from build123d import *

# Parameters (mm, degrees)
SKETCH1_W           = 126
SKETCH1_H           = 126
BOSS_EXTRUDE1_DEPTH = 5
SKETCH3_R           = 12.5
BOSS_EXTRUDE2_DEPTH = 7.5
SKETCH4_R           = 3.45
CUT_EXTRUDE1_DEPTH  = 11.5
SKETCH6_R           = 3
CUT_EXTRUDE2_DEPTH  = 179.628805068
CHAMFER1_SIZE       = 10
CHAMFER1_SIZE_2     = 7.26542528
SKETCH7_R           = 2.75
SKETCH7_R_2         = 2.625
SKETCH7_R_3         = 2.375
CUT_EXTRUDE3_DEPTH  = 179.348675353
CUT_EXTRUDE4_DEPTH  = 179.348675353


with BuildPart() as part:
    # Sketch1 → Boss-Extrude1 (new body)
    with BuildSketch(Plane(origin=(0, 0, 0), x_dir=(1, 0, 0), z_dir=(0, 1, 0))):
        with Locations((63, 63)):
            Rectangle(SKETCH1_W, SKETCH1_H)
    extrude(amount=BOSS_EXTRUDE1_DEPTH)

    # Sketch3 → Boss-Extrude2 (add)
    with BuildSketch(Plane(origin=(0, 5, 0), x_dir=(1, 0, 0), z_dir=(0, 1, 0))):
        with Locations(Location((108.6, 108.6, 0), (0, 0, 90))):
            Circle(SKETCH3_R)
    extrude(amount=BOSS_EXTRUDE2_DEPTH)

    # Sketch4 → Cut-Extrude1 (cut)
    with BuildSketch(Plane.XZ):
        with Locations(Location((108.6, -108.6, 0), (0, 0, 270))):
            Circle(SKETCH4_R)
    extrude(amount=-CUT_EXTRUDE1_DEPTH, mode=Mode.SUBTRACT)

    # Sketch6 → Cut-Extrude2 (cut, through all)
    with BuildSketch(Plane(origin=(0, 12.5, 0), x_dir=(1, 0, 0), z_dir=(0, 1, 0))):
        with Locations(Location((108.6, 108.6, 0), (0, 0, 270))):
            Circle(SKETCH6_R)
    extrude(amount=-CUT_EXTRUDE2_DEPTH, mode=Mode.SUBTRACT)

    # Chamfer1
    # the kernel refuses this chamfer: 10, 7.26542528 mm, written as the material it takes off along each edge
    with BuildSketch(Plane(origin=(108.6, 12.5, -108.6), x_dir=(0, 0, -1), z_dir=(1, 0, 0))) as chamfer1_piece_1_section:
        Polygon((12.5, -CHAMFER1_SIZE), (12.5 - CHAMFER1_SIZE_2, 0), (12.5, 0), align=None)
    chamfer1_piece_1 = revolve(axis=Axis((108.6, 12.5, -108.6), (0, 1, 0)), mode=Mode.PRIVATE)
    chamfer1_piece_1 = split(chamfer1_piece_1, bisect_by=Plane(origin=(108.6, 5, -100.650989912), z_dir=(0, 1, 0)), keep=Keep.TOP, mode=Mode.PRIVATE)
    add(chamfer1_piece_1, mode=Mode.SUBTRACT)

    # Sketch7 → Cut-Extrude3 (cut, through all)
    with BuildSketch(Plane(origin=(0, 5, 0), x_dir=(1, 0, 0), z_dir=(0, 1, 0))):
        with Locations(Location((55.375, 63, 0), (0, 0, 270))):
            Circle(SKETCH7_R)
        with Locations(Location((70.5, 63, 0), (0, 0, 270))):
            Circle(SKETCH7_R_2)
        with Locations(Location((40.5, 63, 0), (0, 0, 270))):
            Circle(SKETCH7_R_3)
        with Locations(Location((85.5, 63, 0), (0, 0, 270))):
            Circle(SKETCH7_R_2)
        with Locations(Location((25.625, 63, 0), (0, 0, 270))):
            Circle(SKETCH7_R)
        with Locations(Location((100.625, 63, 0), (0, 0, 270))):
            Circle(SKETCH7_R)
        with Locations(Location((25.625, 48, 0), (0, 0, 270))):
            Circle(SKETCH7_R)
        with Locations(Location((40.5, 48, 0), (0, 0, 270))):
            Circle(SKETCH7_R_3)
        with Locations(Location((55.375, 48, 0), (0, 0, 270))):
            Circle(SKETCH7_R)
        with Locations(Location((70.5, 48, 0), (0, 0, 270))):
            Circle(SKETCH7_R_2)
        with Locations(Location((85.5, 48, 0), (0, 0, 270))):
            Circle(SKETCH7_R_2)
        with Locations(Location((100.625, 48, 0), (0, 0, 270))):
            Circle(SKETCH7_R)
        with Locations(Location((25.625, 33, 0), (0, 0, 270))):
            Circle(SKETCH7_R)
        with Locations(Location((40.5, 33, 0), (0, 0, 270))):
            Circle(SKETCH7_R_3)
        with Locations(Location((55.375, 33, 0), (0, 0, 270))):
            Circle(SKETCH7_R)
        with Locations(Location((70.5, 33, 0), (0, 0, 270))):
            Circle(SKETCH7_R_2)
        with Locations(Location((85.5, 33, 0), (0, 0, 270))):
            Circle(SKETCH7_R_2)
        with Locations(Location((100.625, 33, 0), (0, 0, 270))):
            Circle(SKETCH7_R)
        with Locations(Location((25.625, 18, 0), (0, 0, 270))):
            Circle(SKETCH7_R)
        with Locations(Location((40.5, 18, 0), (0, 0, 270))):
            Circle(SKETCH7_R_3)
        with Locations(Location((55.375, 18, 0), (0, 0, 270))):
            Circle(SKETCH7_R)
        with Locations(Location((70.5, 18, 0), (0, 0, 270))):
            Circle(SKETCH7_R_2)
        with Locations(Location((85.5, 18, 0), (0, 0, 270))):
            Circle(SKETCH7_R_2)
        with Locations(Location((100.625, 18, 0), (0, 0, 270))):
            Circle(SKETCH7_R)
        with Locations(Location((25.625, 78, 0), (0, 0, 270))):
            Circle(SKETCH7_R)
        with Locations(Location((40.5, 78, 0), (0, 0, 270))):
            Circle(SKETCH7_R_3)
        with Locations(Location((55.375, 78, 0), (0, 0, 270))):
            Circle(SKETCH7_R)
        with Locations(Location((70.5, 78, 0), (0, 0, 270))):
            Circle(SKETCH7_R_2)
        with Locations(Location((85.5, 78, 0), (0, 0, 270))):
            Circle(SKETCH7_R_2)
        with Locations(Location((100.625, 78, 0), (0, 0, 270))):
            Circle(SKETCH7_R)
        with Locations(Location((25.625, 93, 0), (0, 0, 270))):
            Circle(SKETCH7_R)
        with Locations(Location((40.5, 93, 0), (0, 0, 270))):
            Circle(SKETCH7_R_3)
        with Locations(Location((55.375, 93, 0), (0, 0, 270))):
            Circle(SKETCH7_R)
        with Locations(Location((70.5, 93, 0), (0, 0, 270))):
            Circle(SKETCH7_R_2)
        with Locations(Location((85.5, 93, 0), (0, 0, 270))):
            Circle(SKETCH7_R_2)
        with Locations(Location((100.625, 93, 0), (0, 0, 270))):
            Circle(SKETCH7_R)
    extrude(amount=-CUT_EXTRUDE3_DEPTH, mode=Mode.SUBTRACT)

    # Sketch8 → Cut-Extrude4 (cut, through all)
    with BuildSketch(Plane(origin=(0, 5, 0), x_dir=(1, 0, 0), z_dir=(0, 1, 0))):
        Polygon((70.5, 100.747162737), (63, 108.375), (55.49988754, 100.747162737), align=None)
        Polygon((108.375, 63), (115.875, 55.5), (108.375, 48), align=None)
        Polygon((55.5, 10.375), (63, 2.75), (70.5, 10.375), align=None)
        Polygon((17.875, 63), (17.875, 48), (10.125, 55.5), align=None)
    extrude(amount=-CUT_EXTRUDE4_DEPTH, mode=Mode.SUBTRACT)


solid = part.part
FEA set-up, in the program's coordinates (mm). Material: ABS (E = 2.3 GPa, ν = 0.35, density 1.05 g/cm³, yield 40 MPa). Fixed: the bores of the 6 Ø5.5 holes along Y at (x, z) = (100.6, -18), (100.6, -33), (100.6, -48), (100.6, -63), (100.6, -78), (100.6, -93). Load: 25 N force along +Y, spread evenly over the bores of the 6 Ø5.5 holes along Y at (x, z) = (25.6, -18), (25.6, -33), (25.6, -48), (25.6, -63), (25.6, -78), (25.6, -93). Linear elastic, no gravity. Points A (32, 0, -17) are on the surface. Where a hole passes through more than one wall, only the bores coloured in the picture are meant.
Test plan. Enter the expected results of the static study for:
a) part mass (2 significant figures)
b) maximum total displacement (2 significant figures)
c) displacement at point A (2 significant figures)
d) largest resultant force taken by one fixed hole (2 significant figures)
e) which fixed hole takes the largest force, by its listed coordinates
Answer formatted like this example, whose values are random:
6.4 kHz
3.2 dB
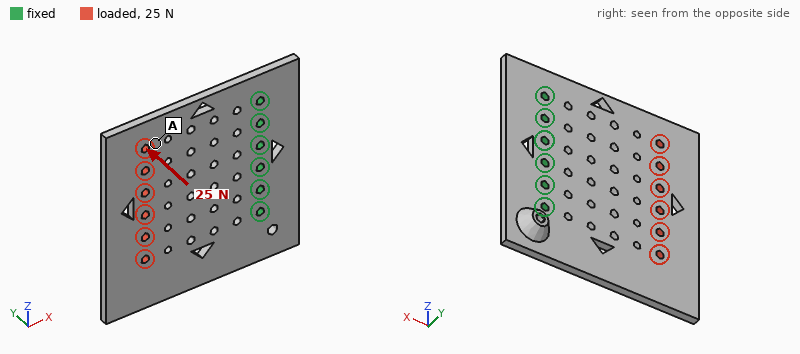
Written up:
79 g
2.0 mm
1.1 mm
6.6 N
(100.6, -33)
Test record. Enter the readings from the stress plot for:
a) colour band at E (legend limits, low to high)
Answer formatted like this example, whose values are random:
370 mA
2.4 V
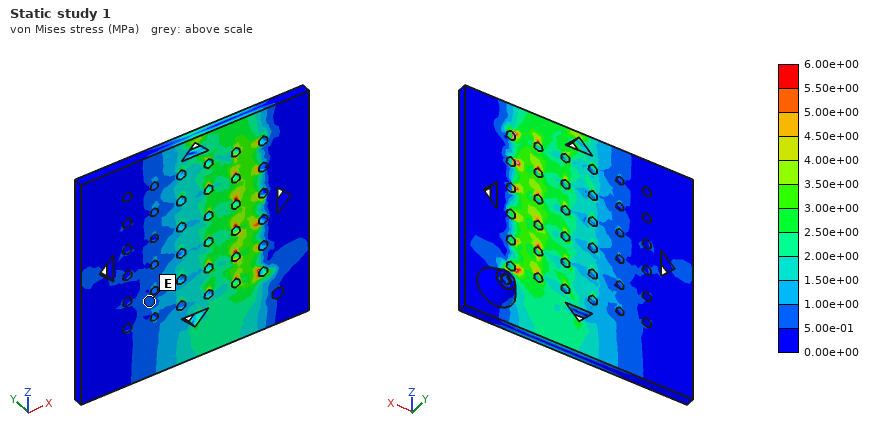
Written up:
5.00e-01 to 1.00e+00 MPa
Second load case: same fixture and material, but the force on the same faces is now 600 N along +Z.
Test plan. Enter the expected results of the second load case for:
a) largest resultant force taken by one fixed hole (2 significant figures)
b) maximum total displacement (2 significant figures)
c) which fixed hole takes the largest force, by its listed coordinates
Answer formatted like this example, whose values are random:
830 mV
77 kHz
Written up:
550 N
0.32 mm
(100.6, -93)
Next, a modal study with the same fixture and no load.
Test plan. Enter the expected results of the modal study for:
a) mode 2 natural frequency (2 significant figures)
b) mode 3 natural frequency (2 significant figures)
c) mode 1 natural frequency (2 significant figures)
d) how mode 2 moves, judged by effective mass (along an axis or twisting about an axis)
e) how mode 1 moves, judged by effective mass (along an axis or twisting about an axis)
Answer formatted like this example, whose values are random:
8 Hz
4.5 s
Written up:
230 Hz
570 Hz
120 Hz
twisting about X
along Y
